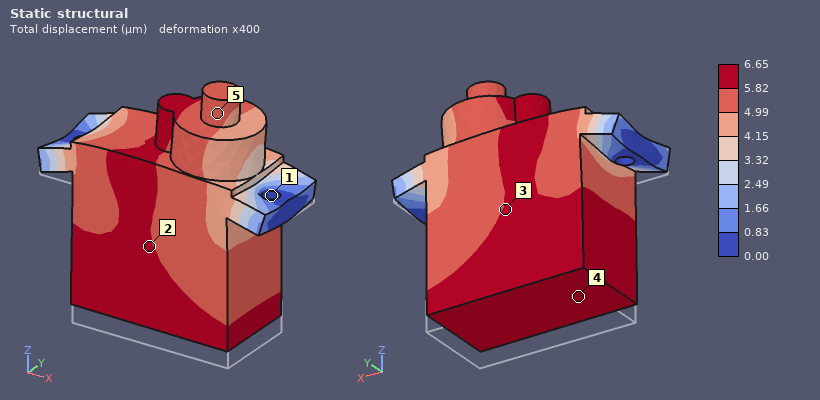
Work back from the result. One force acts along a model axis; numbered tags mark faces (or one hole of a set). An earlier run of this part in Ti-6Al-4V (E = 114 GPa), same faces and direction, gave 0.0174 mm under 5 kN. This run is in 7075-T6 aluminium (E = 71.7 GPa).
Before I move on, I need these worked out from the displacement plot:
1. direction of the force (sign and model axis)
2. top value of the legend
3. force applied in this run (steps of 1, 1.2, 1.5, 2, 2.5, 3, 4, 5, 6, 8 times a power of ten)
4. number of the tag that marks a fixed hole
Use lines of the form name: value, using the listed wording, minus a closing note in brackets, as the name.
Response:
direction of the force: +Z
top value of the legend: 6.65 µm
force applied in this run: 1.2 kN
number of the tag that marks a fixed hole: 1
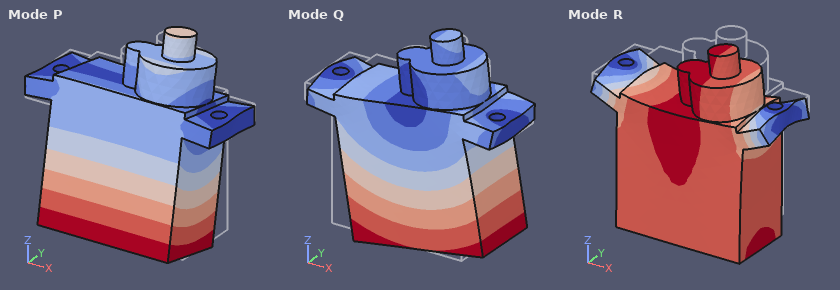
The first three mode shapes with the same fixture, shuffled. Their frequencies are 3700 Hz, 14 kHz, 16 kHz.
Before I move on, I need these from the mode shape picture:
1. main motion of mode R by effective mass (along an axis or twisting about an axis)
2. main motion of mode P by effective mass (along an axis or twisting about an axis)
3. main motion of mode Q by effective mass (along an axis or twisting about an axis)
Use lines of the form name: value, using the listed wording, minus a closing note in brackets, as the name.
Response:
main motion of mode R by effective mass: along Z
main motion of mode P by effective mass: along Y
main motion of mode Q by effective mass: along X
